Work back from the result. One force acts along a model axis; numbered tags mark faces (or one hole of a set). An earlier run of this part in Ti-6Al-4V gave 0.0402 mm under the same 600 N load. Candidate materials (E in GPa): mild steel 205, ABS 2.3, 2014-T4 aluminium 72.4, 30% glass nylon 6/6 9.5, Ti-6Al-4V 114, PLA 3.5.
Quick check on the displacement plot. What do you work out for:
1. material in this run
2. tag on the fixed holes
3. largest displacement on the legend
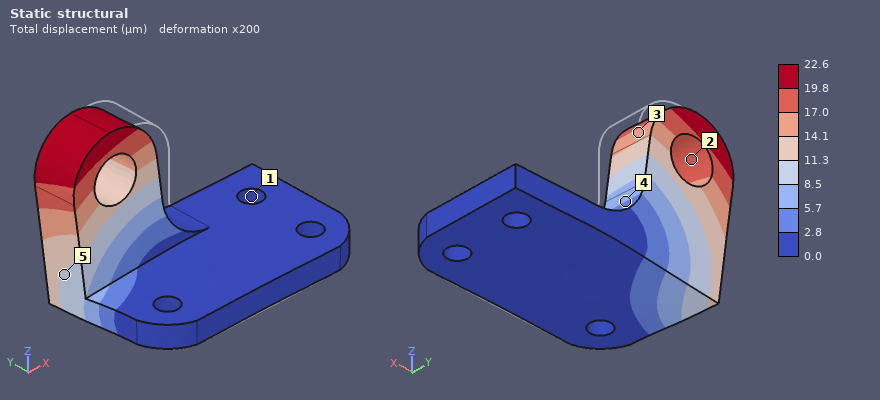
mild steel
1
22.6 µm
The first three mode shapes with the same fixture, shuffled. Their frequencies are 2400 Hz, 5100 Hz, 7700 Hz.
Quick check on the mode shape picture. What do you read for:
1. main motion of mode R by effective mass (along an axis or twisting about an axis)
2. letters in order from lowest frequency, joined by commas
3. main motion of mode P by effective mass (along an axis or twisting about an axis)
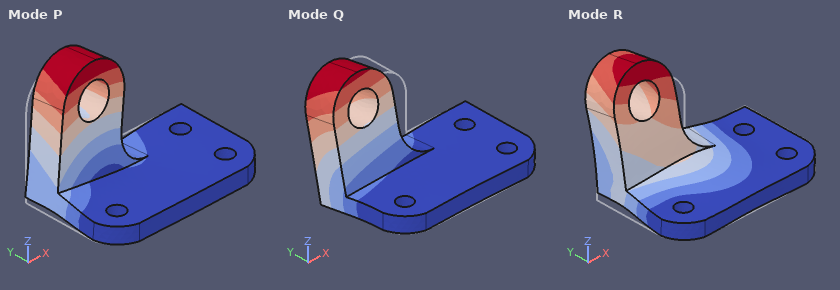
along Z
Q, P, R
along X
